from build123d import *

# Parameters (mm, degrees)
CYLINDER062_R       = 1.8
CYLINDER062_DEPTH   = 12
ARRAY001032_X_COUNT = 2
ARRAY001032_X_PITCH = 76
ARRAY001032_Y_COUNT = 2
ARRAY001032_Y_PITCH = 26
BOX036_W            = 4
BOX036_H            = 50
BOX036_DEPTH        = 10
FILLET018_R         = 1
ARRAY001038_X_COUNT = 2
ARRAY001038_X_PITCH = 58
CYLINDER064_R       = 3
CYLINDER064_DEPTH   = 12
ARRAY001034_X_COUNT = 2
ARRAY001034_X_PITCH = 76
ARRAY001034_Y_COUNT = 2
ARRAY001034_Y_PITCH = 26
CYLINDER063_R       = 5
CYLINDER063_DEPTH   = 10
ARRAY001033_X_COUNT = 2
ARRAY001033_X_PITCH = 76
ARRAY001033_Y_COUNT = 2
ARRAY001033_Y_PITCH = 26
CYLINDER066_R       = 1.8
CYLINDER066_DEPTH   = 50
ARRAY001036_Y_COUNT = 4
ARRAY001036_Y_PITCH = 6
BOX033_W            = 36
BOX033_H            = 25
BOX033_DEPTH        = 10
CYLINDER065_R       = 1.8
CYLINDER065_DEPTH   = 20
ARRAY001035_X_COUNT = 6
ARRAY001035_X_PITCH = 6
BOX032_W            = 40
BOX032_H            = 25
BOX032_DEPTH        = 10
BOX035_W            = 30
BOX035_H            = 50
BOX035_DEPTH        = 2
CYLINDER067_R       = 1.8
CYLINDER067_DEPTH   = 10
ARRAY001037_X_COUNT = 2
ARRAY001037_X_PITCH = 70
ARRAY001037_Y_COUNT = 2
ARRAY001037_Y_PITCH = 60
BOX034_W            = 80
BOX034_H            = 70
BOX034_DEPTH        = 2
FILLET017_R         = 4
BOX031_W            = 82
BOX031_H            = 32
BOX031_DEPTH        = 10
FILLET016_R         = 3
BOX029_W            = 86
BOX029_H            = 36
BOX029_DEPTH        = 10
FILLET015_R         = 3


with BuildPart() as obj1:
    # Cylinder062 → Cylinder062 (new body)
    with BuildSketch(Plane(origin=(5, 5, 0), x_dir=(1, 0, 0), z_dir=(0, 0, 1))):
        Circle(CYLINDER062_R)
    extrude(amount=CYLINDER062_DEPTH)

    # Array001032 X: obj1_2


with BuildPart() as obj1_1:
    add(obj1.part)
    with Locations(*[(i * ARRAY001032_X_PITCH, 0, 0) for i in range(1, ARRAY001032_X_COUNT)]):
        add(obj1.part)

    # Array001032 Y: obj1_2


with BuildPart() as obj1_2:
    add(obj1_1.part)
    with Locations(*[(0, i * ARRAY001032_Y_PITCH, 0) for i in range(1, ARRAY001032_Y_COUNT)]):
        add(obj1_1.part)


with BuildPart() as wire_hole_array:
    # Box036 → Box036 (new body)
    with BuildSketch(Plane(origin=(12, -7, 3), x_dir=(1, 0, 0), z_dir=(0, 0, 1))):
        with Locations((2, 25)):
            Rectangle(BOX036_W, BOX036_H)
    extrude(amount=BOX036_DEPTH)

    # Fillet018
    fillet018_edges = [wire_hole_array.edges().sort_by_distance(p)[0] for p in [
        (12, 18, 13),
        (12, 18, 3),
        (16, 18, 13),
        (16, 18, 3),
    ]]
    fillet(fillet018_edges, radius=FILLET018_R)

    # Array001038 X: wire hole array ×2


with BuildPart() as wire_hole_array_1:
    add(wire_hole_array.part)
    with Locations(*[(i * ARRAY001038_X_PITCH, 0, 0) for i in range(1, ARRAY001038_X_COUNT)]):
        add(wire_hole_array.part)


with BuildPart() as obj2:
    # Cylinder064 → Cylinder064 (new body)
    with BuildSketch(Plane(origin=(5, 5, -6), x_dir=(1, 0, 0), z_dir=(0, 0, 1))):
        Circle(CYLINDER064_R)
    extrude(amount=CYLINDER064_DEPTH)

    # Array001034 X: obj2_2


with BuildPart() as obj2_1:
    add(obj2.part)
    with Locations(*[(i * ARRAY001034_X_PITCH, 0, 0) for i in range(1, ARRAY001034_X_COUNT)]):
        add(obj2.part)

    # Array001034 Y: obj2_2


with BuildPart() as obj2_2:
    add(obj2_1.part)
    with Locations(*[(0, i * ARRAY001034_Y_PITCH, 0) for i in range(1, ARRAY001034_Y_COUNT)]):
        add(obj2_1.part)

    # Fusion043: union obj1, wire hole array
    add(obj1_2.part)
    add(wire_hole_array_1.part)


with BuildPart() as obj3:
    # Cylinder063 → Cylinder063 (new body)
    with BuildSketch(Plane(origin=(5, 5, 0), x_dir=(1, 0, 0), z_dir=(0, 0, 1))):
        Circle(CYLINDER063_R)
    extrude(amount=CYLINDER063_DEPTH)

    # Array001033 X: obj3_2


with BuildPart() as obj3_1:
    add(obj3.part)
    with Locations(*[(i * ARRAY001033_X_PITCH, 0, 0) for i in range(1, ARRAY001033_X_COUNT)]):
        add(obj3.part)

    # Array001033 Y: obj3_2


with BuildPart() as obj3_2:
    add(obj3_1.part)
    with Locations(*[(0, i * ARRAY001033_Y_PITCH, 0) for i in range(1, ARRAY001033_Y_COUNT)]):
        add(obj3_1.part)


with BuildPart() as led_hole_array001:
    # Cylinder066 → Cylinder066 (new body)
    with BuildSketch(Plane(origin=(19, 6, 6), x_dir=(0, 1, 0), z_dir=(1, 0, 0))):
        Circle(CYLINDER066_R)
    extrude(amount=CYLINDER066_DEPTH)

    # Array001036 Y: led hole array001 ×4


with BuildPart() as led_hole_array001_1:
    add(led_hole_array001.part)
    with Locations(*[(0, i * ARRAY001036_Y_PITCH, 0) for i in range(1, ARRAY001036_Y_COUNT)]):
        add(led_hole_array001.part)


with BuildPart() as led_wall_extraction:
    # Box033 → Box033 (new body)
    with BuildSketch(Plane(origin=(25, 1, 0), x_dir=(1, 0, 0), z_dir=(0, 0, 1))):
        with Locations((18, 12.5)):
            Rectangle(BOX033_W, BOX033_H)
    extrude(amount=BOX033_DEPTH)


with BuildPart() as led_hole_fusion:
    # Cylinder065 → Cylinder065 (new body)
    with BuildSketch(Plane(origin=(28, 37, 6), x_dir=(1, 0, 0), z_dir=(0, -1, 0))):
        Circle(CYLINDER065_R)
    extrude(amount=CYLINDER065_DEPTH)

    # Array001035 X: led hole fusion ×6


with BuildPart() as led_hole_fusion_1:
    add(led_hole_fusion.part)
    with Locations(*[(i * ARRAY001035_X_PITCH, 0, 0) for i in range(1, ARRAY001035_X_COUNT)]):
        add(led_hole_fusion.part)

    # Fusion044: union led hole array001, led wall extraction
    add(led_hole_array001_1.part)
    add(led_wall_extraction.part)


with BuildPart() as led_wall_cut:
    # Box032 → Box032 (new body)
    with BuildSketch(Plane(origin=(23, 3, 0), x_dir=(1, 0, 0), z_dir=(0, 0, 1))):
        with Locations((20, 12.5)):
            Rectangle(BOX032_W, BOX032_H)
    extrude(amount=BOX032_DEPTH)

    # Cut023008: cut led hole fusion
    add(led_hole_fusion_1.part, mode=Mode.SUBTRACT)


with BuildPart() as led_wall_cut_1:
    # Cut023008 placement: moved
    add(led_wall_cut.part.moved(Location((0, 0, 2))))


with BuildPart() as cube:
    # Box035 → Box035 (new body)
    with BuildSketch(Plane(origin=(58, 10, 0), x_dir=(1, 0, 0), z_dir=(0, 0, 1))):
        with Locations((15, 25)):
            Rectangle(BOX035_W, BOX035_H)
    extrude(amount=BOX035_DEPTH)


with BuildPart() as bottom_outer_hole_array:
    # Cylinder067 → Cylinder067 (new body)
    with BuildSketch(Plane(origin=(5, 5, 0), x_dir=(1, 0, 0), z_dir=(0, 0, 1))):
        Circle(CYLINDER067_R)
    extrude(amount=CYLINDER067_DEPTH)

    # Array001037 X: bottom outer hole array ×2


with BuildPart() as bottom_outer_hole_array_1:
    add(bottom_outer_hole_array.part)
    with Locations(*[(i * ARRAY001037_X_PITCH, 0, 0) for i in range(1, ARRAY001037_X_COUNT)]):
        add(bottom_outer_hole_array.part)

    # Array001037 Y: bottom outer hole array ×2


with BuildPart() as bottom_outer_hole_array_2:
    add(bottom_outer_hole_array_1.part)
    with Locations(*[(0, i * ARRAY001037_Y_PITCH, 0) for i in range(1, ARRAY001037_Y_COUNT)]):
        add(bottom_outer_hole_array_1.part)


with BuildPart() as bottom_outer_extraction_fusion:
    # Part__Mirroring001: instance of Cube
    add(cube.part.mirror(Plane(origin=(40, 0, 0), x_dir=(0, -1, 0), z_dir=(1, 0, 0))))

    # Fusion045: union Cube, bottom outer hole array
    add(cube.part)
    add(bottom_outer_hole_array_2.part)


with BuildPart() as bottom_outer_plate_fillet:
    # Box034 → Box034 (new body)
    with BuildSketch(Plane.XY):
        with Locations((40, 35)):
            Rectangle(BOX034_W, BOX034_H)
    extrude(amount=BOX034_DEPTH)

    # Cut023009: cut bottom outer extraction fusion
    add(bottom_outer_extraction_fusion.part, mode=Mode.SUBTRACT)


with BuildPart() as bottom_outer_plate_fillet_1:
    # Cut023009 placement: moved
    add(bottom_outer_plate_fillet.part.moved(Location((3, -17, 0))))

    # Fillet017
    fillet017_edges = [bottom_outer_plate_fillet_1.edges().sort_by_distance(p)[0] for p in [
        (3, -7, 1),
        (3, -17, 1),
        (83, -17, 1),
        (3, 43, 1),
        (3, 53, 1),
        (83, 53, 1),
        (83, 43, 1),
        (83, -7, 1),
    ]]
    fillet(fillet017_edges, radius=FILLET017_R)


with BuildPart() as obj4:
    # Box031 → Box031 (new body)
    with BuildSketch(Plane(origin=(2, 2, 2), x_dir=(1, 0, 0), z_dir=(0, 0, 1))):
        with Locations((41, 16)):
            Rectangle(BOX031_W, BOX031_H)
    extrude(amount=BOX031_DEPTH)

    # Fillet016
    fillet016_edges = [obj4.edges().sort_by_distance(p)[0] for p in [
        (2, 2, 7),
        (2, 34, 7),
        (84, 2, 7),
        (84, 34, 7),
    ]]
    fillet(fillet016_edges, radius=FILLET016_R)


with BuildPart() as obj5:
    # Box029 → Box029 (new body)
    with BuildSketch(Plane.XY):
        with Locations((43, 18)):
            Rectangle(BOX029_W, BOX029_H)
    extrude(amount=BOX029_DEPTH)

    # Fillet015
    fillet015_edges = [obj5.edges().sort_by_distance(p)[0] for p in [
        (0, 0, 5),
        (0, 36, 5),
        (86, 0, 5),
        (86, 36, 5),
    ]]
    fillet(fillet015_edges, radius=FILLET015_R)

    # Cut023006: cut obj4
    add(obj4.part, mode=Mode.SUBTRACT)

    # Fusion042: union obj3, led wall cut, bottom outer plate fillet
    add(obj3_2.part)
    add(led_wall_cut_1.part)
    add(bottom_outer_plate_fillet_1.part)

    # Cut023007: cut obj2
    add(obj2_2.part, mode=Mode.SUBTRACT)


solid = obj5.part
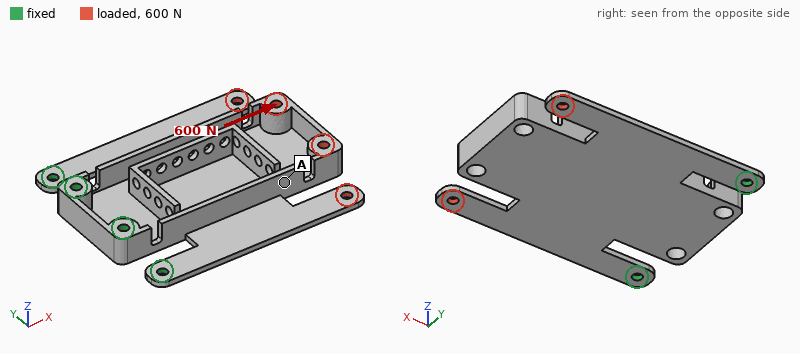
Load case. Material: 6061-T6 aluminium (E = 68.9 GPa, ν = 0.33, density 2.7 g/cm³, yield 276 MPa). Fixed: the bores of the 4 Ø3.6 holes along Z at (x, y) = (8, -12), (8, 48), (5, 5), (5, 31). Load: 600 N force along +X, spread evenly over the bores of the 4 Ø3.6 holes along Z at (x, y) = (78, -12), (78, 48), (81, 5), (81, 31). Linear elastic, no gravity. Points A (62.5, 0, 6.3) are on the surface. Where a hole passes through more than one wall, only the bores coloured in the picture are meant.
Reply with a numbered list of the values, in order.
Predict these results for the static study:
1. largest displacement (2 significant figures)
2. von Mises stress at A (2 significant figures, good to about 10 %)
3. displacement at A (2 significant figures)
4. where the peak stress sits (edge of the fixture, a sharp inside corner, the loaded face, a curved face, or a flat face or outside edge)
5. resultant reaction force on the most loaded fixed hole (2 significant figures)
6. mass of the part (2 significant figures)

1. 0.89 mm
2. 20 MPa
3. 0.46 mm
4. a curved face
5. 230 N
6. 44 g
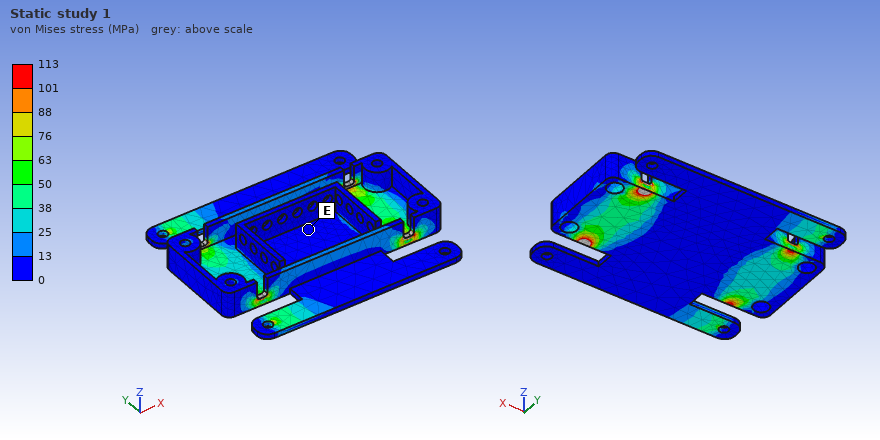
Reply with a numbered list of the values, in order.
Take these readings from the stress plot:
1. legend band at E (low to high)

1. 0 to 13 MPa
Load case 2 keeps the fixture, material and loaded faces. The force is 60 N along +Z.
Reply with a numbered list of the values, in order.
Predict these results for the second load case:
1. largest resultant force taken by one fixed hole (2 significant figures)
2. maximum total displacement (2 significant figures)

1. 150 N
2. 1.1 mm
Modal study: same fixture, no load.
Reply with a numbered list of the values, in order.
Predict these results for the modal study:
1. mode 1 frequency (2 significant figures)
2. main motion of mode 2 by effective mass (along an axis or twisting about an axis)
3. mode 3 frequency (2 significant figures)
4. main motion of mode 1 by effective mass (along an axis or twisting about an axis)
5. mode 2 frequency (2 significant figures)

1. 340 Hz
2. twisting about X
3. 1900 Hz
4. along Z
5. 820 Hz
